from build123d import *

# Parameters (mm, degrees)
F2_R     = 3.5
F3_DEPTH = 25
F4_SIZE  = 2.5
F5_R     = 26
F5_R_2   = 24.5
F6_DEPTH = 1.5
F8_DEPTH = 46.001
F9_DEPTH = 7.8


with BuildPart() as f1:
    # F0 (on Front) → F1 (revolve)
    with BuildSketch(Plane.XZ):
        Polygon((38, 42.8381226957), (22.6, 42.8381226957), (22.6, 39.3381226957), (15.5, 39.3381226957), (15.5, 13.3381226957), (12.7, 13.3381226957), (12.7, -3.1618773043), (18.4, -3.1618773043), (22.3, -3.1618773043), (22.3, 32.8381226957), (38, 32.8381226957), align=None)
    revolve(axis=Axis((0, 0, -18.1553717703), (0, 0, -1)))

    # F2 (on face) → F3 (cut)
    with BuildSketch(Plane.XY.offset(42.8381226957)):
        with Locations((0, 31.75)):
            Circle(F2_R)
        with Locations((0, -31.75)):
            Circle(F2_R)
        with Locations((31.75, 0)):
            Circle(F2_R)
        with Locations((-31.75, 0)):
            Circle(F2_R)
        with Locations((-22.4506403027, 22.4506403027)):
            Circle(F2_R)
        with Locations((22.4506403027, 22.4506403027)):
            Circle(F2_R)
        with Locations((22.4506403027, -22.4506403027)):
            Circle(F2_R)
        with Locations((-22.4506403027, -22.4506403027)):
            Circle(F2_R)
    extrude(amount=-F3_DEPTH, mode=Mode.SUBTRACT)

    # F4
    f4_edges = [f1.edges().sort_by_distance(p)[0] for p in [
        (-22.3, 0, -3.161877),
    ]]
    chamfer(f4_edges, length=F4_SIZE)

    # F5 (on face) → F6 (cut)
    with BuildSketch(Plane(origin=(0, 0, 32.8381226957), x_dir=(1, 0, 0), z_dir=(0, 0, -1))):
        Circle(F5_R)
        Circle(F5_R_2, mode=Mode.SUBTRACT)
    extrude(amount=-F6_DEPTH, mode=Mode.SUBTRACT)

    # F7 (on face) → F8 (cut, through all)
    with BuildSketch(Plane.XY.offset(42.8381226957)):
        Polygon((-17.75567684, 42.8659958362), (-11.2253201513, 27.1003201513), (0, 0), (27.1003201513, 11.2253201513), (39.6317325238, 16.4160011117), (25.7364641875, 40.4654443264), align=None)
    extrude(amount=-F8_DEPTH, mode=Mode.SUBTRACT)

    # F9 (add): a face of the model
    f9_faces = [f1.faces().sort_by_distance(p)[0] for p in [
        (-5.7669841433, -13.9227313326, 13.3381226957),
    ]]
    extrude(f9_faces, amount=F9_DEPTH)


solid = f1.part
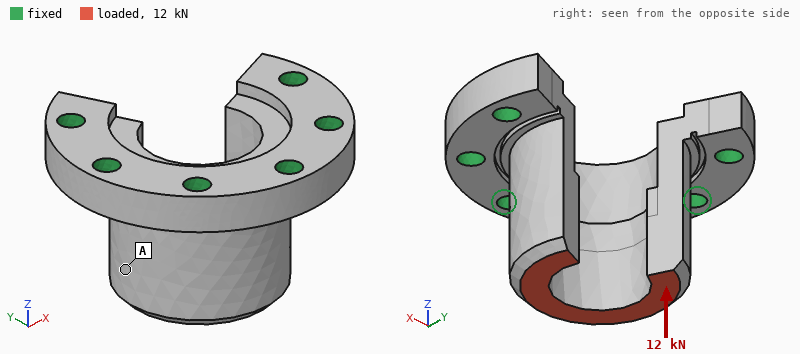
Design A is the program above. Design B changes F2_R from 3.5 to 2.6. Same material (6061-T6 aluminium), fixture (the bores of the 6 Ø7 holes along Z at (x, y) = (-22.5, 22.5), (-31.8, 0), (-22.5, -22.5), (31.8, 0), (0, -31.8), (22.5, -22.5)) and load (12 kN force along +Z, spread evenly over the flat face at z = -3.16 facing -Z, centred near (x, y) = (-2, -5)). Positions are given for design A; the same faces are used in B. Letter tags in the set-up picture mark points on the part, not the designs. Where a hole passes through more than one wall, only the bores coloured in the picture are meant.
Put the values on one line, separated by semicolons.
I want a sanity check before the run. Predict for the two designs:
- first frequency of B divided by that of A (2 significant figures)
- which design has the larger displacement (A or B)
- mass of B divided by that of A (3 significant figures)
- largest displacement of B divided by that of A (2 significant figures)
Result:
0.98; B; 1.02; 1.1
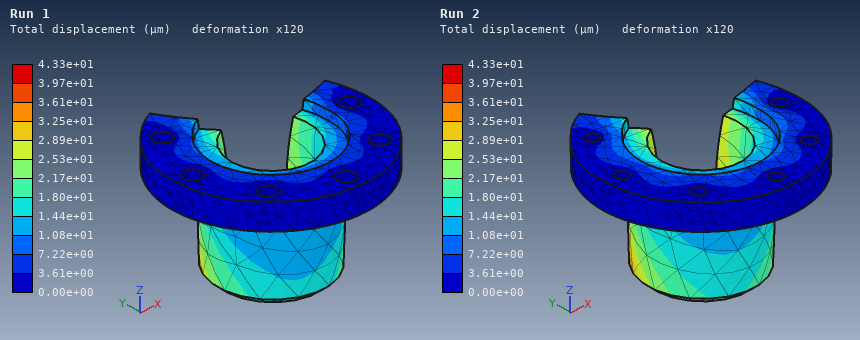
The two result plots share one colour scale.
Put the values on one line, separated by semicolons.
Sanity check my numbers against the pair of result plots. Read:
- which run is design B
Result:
Run 2
